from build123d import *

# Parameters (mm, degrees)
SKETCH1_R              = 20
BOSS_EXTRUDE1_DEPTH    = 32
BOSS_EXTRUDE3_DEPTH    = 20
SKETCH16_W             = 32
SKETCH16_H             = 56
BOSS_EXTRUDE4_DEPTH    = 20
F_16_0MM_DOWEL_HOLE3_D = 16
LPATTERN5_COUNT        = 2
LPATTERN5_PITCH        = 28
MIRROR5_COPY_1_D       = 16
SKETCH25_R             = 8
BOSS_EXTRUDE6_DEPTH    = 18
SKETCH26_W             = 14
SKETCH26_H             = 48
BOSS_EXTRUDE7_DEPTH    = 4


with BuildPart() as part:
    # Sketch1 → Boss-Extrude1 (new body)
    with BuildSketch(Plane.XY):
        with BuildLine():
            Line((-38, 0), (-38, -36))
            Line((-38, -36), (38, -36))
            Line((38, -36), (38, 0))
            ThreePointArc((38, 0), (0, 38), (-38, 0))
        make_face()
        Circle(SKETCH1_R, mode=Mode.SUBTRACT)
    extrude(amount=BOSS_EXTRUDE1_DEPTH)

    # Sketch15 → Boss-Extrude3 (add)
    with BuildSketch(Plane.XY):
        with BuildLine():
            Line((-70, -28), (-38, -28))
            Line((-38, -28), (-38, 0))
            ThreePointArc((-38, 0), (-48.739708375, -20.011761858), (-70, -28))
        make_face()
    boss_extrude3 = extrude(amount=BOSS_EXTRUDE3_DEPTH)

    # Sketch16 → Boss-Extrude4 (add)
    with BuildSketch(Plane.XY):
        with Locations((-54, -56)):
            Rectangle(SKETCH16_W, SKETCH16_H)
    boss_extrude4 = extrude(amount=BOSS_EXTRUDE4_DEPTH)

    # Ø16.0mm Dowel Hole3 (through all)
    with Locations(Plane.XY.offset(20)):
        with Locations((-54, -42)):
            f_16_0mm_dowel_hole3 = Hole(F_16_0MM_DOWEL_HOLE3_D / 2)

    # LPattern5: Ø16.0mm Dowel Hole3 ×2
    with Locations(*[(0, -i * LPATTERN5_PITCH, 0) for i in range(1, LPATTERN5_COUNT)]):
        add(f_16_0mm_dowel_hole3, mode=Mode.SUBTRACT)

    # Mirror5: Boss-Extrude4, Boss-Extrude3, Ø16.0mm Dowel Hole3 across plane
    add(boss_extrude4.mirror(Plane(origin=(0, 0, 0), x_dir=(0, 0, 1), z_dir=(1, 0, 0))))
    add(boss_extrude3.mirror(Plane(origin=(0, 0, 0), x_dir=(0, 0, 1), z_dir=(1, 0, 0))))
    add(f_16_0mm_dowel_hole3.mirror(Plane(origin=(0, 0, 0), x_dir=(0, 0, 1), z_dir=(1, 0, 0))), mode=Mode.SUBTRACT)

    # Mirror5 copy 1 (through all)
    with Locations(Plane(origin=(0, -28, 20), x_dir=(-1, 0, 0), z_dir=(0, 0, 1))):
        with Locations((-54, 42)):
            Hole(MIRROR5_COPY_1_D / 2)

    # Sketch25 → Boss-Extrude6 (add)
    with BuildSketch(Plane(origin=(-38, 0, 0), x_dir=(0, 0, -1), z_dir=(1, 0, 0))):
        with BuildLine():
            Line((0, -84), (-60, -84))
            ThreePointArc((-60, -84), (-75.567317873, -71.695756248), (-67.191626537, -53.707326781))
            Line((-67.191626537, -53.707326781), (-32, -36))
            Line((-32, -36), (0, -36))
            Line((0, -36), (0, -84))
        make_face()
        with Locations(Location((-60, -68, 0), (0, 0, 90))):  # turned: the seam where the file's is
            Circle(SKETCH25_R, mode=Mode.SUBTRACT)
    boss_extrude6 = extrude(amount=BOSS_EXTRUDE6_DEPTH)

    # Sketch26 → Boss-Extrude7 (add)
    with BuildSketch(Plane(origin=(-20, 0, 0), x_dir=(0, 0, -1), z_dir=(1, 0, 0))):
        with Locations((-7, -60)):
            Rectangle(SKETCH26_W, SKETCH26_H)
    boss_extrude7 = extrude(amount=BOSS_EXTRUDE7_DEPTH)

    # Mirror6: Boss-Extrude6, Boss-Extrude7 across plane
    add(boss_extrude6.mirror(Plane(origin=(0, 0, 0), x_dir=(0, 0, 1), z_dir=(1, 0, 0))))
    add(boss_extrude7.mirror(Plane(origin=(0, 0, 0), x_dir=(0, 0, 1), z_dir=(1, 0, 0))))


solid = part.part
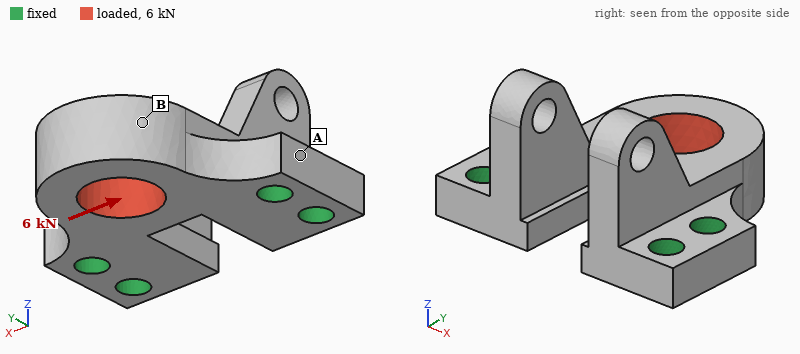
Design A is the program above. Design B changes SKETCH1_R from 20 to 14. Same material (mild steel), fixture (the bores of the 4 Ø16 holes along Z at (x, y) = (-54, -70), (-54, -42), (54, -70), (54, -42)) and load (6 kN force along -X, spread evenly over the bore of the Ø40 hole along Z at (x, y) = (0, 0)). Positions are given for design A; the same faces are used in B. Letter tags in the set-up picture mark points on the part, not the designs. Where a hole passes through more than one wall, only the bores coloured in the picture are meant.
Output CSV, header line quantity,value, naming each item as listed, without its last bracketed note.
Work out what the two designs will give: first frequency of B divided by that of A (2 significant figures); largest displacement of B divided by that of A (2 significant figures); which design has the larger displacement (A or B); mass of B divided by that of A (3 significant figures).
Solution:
quantity,value
first frequency of B divided by that of A,0.96
largest displacement of B divided by that of A,0.60
which design has the larger displacement,A
mass of B divided by that of A,1.07
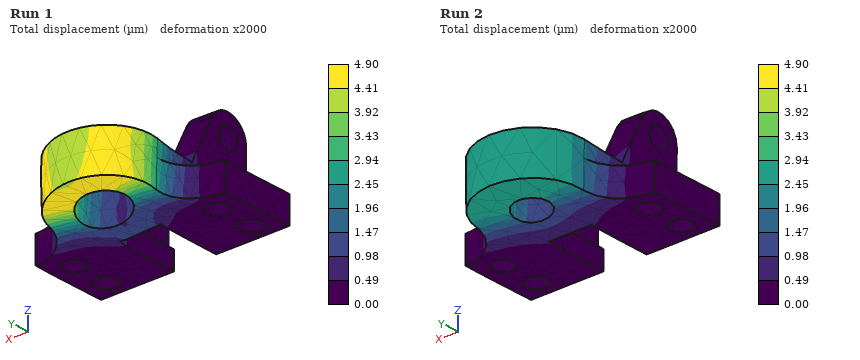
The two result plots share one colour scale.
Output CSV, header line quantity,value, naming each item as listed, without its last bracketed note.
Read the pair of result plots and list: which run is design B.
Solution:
quantity,value
which run is design B,Run 2
